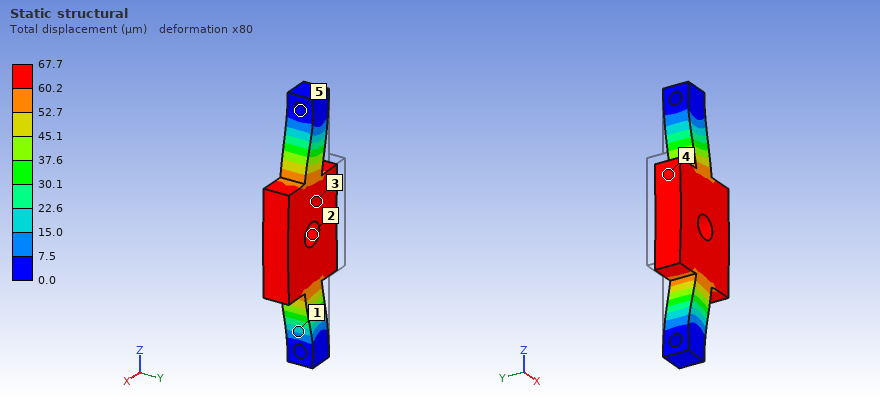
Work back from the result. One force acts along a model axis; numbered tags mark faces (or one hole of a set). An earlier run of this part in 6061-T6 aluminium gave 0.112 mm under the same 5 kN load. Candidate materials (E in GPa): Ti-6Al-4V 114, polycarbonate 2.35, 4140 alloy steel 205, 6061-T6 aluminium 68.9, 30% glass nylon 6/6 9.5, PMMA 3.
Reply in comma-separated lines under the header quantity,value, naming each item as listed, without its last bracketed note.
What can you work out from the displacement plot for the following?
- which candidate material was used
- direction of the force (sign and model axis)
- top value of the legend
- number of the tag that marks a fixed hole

quantity,value
which candidate material was used,Ti-6Al-4V
direction of the force,+X
top value of the legend,67.7 µm
number of the tag that marks a fixed hole,5
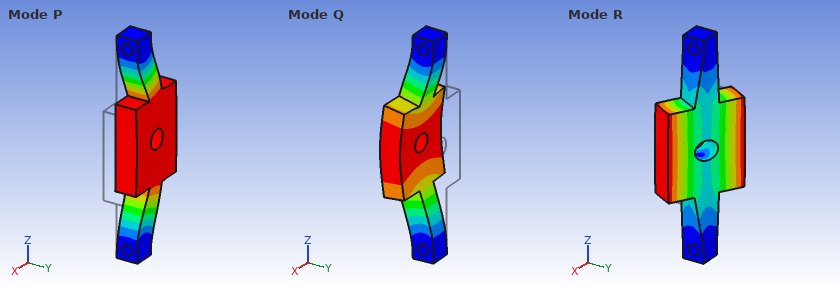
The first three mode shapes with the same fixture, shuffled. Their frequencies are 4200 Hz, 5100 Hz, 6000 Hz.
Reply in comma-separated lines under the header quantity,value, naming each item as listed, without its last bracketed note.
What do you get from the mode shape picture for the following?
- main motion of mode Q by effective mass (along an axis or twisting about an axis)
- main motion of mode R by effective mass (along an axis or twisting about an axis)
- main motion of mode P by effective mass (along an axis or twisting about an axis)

quantity,value
main motion of mode Q by effective mass,along Y
main motion of mode R by effective mass,twisting about Z
main motion of mode P by effective mass,along X
